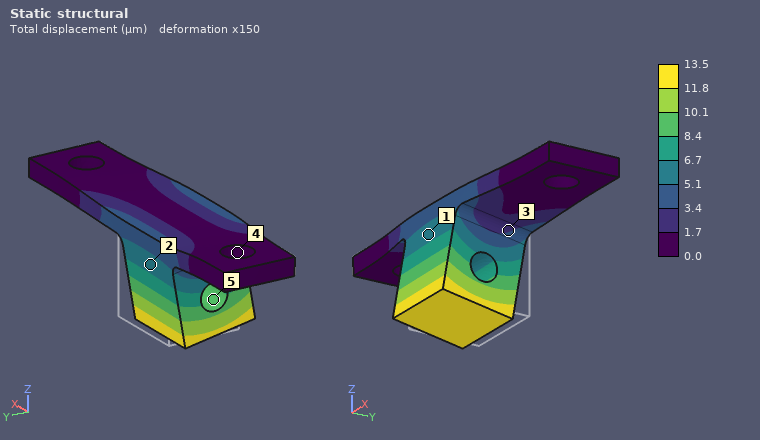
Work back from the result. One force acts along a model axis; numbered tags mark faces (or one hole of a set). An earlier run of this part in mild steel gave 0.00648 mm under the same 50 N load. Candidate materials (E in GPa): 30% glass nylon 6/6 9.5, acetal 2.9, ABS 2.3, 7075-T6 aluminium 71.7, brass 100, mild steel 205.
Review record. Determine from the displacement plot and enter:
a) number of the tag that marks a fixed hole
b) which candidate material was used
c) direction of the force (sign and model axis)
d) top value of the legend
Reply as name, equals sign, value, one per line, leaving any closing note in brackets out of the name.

number of the tag that marks a fixed hole = 4
which candidate material was used = brass
direction of the force = -Y
top value of the legend = 13.5 µm
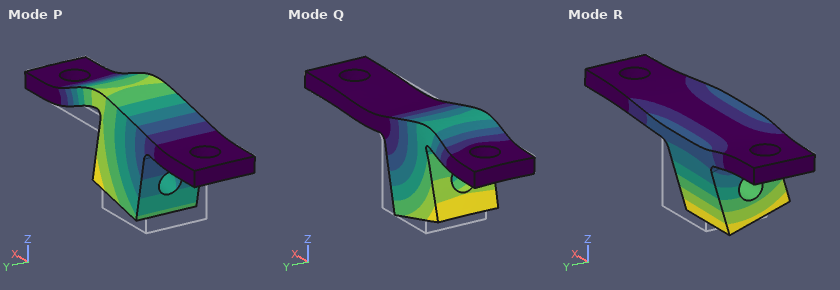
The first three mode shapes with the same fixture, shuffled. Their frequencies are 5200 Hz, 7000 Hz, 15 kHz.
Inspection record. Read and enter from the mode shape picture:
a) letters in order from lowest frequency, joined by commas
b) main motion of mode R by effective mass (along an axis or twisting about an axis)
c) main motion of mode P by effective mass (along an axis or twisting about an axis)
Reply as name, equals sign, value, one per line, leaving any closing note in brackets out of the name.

letters in order from lowest frequency, joined by commas = R, P, Q
main motion of mode R by effective mass = along Y
main motion of mode P by effective mass = along Z
